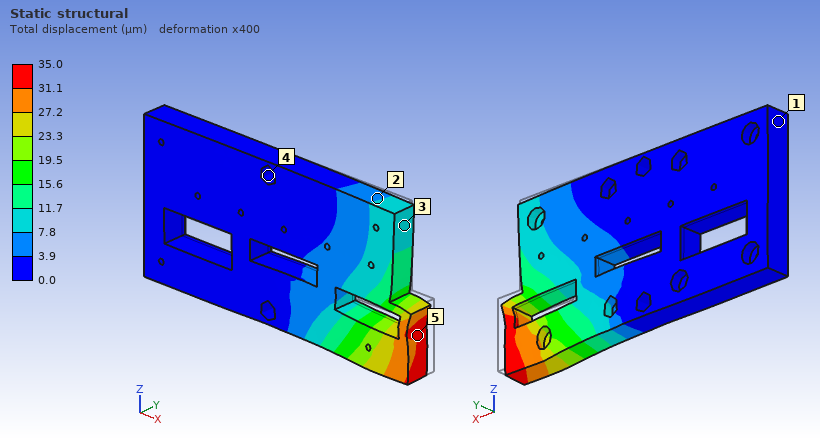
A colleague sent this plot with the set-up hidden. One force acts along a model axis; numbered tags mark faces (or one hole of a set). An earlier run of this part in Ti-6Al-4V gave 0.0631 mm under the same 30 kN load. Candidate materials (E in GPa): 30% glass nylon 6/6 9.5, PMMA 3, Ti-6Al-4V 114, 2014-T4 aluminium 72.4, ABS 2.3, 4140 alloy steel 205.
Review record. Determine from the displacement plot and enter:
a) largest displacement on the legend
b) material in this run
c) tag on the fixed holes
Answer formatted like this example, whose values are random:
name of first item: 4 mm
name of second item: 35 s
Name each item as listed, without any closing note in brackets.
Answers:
largest displacement on the legend: 35.0 µm
material in this run: 4140 alloy steel
tag on the fixed holes: 4
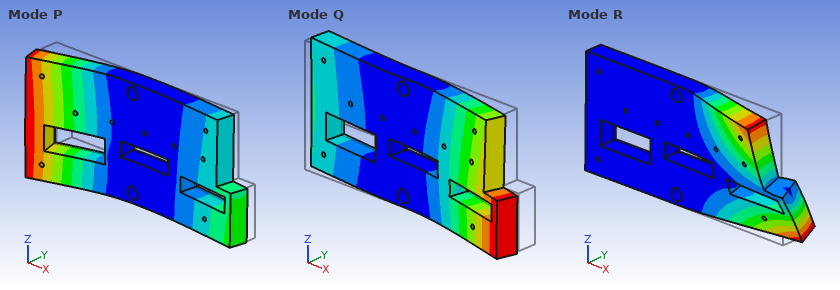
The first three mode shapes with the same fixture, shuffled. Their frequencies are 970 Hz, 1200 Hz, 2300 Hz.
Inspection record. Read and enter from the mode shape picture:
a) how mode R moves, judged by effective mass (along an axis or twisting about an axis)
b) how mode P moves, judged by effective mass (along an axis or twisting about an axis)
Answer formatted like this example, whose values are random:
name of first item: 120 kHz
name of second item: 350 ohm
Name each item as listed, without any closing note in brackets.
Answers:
how mode R moves, judged by effective mass: twisting about X
how mode P moves, judged by effective mass: along Y
